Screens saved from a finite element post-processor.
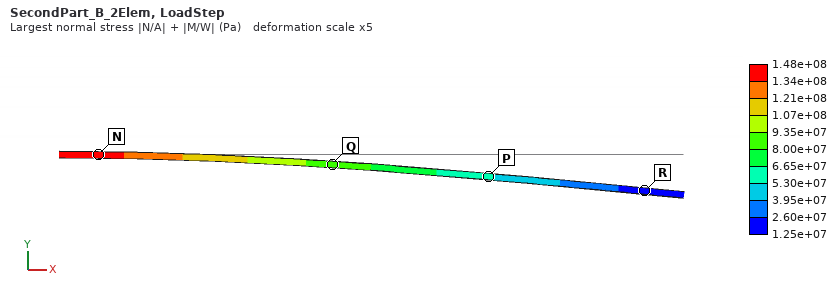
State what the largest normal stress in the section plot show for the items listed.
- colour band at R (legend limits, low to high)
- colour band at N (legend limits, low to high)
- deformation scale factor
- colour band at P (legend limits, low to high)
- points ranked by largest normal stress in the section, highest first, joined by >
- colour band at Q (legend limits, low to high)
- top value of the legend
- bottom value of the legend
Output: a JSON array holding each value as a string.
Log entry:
["1.25e+07 to 2.60e+07 Pa", "1.34e+08 to 1.48e+08 Pa", "5", "5.30e+07 to 6.65e+07 Pa", "N > Q > P > R", "8.00e+07 to 9.35e+07 Pa", "1.48e+08 Pa", "1.25e+07 Pa"]
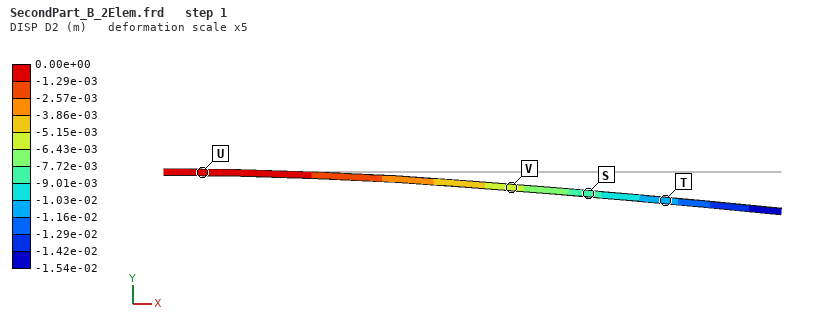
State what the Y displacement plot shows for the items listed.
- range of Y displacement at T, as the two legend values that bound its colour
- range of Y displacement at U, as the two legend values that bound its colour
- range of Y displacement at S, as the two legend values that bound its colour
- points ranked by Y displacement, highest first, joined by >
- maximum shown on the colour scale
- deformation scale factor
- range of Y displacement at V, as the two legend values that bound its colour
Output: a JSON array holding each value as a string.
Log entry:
["-1.16e-02 to -1.03e-02 m", "-1.29e-03 to 0.00e+00 m", "-9.01e-03 to -7.72e-03 m", "U > V > S > T", "0.00e+00 m", "5", "-6.43e-03 to -5.15e-03 m"]
